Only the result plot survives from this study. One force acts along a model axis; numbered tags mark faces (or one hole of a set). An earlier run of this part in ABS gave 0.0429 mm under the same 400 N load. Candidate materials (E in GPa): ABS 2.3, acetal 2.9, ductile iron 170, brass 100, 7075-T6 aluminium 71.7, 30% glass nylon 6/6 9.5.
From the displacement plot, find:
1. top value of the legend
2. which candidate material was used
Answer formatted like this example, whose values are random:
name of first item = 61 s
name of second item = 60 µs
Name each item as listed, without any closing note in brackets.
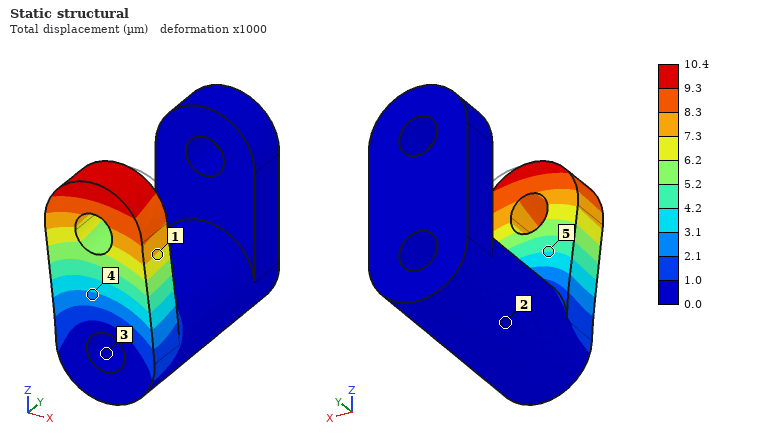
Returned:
top value of the legend = 10.4 µm
which candidate material was used = 30% glass nylon 6/6
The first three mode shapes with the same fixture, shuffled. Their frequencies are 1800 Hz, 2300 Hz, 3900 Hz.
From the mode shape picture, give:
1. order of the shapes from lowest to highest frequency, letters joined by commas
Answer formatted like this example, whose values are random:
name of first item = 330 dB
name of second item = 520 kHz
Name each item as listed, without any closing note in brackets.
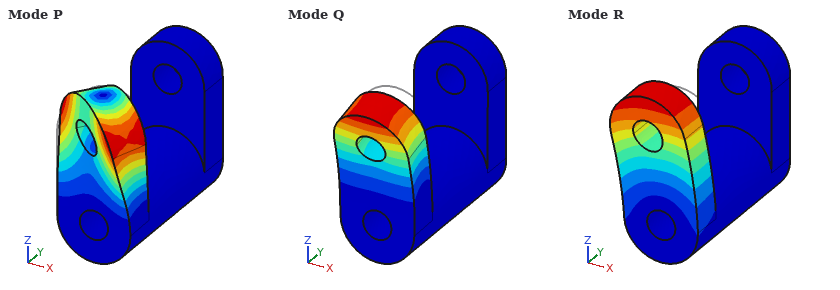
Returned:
order of the shapes from lowest to highest frequency, letters joined by commas = Q, R, P
